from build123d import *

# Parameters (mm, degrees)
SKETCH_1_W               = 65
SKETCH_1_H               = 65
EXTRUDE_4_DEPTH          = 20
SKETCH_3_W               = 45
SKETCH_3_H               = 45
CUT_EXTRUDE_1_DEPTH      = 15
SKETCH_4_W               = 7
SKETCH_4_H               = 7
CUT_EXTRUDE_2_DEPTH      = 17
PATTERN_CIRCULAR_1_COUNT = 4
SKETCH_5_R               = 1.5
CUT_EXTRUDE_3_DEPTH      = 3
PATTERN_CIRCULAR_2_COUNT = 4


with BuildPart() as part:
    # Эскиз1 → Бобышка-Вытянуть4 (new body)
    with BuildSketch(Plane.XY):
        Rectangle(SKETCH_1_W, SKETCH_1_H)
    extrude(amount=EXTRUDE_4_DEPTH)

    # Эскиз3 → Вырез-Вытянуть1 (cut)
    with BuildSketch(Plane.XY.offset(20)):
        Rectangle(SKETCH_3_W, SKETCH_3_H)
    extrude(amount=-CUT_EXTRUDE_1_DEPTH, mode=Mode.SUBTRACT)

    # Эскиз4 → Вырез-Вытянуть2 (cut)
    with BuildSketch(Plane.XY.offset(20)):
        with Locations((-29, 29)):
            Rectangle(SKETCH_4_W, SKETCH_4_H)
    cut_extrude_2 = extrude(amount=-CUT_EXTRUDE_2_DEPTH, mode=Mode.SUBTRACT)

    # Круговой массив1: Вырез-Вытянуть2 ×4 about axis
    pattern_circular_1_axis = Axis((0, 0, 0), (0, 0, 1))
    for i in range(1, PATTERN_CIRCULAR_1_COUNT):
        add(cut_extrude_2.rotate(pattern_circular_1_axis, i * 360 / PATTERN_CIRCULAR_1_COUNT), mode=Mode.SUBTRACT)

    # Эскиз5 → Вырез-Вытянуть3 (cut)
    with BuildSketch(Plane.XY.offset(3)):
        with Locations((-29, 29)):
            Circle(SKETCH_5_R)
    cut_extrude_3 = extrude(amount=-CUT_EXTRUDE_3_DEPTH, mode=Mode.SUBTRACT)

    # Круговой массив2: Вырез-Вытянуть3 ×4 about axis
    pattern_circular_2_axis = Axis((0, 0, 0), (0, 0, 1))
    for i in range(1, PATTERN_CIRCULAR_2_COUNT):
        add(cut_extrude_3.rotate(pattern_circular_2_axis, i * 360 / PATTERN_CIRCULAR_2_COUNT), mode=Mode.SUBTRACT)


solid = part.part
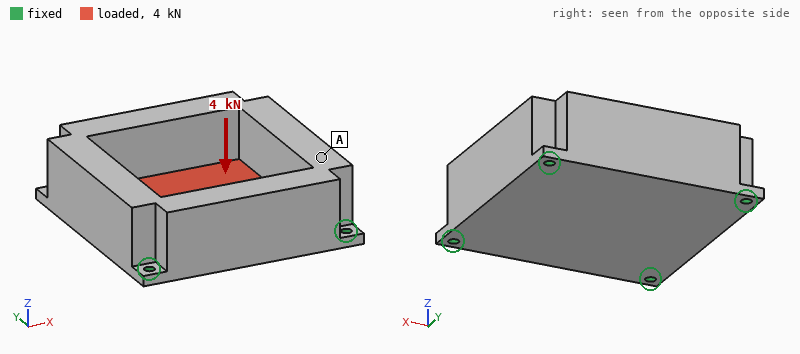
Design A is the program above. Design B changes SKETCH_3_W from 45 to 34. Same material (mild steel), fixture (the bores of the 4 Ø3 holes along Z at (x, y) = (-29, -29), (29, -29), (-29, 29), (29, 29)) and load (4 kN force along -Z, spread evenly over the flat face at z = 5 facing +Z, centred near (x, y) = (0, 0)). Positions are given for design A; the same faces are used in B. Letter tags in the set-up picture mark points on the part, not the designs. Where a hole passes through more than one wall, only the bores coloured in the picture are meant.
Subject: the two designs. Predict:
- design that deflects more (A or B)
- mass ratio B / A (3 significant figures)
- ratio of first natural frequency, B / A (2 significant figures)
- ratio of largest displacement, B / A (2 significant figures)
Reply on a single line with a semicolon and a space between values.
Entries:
A; 1.15; 0.97; 0.84
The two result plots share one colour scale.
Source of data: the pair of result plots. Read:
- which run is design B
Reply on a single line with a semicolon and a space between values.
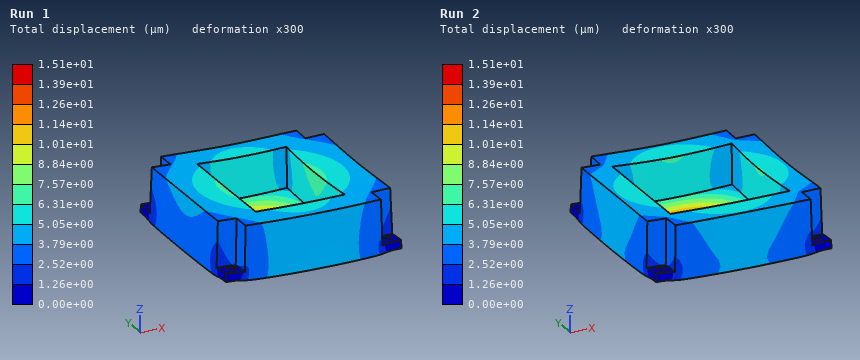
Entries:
Run 1
